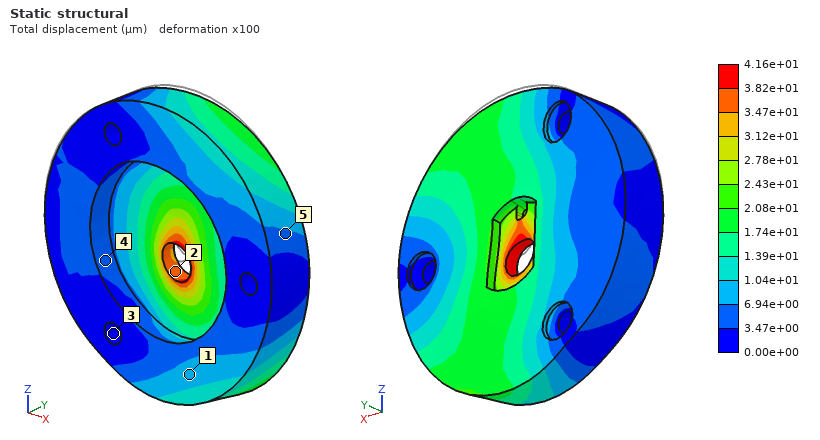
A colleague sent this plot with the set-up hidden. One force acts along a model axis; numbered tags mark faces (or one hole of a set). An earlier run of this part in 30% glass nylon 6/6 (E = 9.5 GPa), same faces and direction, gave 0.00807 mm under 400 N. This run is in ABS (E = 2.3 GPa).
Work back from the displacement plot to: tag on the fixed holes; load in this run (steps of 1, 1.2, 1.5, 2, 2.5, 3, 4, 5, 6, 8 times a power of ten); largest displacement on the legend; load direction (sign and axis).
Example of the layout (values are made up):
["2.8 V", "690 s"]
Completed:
["3", "500 N", "4.16e+01 µm", "-Z"]
